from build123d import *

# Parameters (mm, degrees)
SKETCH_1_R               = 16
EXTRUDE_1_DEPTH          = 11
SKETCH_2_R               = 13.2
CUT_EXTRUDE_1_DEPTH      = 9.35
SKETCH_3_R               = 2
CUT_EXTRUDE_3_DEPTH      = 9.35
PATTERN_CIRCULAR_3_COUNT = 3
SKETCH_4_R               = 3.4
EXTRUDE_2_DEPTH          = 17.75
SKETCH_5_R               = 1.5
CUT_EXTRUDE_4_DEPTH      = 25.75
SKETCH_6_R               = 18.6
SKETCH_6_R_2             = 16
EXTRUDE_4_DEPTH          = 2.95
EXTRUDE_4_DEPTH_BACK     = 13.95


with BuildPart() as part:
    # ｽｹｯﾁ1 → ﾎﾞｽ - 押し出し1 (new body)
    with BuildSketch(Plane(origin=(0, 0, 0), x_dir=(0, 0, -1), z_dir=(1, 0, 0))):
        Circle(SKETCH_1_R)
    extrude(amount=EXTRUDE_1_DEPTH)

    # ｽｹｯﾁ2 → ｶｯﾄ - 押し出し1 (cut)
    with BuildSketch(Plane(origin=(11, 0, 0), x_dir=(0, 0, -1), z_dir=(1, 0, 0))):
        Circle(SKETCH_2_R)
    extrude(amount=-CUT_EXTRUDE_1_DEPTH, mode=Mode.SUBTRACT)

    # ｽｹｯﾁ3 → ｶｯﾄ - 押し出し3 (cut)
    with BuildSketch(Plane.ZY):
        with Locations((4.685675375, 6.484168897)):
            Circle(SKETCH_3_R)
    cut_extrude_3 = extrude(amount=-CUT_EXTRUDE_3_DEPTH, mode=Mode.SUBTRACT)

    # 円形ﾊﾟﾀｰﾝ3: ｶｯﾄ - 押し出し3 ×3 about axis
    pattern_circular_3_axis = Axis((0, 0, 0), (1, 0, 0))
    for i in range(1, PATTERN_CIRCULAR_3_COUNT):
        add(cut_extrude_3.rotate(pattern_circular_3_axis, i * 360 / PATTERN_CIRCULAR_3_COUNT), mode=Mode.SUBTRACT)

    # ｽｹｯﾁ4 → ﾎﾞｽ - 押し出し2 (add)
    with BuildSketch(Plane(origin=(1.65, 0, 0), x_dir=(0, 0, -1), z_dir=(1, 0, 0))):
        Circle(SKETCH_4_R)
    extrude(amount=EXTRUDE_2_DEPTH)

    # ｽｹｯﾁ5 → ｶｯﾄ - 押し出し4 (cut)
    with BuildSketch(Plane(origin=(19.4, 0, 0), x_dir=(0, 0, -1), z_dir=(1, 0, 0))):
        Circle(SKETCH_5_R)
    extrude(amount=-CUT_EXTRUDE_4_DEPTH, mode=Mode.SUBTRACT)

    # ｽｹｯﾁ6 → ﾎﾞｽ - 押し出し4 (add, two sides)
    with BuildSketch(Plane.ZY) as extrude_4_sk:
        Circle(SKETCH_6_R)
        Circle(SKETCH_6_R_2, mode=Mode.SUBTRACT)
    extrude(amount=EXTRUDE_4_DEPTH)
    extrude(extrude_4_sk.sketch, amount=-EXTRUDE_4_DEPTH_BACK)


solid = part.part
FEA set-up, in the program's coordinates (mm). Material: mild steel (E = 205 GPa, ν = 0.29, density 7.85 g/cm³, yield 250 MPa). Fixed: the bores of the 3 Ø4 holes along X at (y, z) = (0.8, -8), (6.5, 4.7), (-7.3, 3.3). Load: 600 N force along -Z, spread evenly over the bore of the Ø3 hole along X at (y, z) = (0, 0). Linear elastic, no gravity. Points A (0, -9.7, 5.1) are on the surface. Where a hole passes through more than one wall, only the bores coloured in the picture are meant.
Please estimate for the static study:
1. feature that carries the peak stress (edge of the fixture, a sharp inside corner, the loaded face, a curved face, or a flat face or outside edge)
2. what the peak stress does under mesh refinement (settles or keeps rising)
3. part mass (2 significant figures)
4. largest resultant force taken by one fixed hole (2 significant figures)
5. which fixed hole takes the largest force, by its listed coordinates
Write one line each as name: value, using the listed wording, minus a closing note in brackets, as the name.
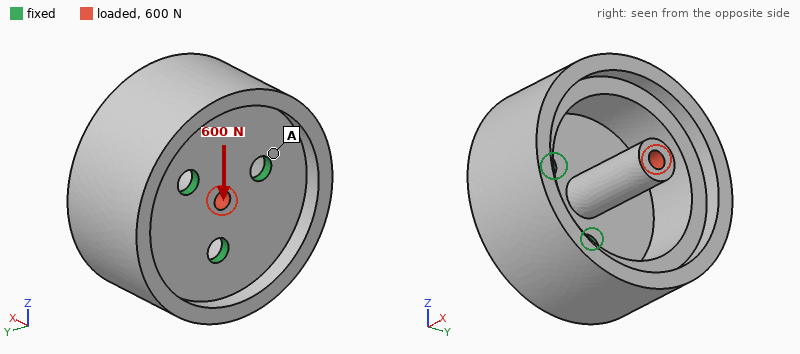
feature that carries the peak stress: edge of the fixture
what the peak stress does under mesh refinement: keeps rising
part mass: 70 g
largest resultant force taken by one fixed hole: 620 N
which fixed hole takes the largest force, by its listed coordinates: (0.8, -8)
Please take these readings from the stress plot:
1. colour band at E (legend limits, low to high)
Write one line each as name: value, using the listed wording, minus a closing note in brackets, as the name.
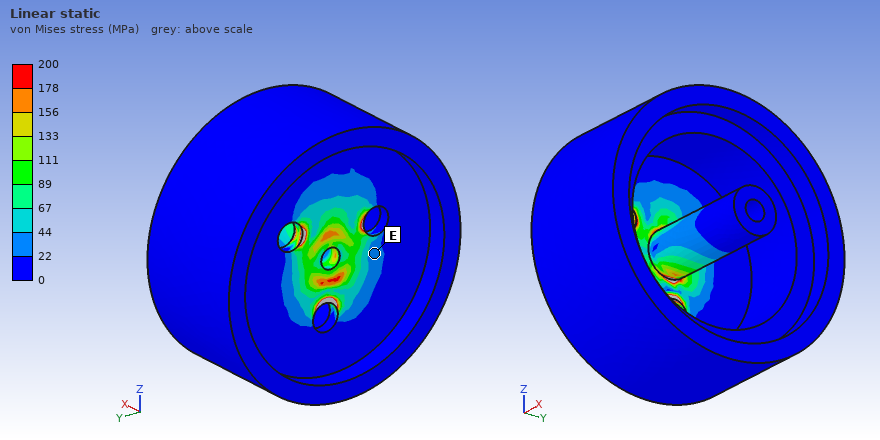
colour band at E: 22 to 44 MPa
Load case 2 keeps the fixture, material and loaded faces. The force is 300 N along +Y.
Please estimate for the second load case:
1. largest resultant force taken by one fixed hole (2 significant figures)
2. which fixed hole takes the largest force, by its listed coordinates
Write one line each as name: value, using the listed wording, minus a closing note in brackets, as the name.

largest resultant force taken by one fixed hole: 290 N
which fixed hole takes the largest force, by its listed coordinates: (-7.3, 3.3)
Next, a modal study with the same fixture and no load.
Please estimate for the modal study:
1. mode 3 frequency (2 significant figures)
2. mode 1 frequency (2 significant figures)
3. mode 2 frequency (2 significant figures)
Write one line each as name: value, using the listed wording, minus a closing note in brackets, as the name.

mode 3 frequency: 9300 Hz
mode 1 frequency: 6100 Hz
mode 2 frequency: 6100 Hz
